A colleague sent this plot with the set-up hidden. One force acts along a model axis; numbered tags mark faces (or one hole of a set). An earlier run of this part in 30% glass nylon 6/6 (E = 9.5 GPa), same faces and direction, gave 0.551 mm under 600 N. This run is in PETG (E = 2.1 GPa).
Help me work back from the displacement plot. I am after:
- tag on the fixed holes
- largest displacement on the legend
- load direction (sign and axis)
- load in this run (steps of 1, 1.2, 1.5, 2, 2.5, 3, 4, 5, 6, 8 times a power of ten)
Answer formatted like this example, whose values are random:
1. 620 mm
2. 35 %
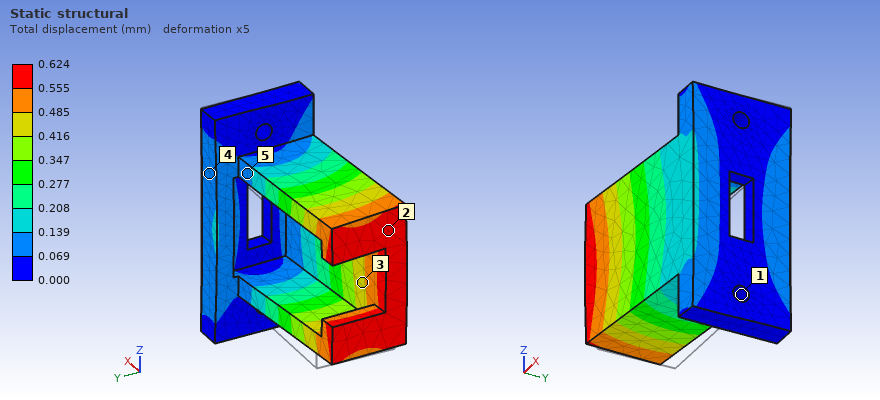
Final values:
1. 1
2. 0.624 mm
3. -Y
4. 150 N
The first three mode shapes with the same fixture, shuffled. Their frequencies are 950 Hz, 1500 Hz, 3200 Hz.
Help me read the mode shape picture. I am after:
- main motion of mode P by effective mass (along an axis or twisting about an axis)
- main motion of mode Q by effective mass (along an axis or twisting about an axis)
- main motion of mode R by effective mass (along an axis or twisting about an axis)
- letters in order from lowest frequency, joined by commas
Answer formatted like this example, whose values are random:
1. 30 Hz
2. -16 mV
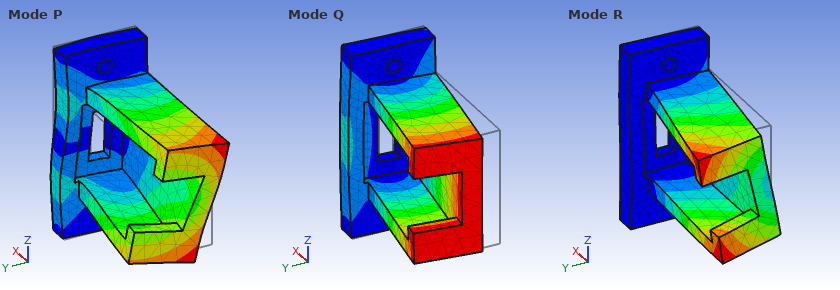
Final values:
1. along Z
2. along Y
3. along Z
4. Q, R, P
